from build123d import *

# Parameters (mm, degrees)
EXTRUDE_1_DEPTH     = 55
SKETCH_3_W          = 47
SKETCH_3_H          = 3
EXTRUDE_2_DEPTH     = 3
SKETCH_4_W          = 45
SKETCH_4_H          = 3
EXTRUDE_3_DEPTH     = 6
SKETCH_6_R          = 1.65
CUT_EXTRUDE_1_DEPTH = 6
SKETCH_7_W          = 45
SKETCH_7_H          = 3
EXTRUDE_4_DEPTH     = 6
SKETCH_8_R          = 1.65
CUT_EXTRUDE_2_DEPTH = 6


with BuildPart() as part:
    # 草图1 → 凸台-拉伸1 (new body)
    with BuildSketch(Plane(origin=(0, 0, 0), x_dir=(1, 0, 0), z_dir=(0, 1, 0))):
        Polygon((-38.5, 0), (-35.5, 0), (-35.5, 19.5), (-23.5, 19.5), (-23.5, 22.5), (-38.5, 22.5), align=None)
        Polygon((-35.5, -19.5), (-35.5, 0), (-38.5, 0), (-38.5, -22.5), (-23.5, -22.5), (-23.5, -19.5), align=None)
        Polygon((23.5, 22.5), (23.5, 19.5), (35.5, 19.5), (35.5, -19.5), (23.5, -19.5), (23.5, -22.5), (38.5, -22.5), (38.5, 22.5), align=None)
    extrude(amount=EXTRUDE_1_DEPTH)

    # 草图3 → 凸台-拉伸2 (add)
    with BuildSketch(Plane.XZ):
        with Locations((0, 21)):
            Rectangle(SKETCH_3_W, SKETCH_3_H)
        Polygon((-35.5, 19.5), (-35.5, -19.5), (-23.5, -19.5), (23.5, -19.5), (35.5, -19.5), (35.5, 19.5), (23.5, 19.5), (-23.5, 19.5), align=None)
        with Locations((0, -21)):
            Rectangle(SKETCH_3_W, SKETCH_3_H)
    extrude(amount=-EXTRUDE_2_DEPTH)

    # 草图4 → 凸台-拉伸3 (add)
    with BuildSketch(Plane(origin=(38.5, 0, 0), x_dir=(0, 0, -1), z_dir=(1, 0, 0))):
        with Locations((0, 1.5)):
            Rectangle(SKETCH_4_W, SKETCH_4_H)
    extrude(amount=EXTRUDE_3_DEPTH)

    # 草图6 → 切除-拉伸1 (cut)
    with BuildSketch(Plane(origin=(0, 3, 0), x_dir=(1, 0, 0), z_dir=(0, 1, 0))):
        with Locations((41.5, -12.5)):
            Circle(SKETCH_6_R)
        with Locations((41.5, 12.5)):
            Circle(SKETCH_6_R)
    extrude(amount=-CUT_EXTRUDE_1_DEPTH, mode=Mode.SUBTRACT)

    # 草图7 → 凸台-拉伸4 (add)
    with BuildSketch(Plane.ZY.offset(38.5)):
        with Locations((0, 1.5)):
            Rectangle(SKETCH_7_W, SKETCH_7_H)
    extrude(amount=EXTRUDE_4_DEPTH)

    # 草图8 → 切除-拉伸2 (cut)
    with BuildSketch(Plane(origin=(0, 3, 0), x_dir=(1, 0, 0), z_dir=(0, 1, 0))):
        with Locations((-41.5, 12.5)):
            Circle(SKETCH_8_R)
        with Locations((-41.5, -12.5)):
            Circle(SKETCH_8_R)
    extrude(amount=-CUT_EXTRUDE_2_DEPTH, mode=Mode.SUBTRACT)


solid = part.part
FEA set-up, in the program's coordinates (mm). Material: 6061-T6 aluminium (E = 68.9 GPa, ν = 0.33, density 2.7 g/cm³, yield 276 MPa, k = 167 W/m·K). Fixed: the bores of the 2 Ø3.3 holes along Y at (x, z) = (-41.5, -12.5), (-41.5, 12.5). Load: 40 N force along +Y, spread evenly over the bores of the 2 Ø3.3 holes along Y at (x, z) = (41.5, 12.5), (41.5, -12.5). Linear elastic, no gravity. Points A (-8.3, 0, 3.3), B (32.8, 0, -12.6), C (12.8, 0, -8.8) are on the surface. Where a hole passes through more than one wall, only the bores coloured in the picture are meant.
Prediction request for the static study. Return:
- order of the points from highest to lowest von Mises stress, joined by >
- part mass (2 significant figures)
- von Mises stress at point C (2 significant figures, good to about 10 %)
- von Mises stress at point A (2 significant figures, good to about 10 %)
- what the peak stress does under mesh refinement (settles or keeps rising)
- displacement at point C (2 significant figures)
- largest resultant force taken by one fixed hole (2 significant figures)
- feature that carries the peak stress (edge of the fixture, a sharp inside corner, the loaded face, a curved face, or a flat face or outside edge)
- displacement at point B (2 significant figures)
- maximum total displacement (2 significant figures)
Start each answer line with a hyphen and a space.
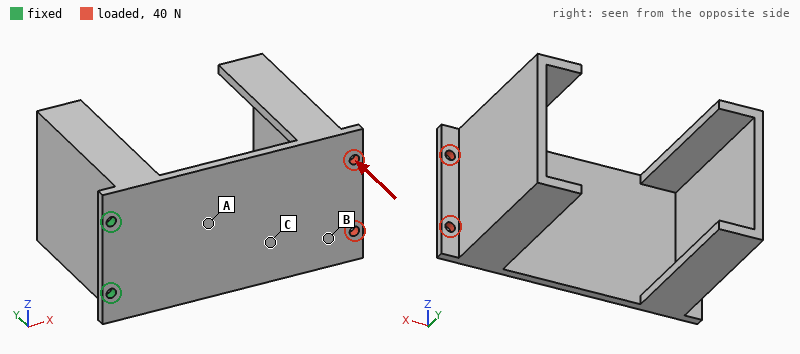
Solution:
- A > C > B
- 90 g
- 17 MPa
- 28 MPa
- keeps rising
- 0.45 mm
- 33 N
- edge of the fixture
- 0.77 mm
- 1.3 mm
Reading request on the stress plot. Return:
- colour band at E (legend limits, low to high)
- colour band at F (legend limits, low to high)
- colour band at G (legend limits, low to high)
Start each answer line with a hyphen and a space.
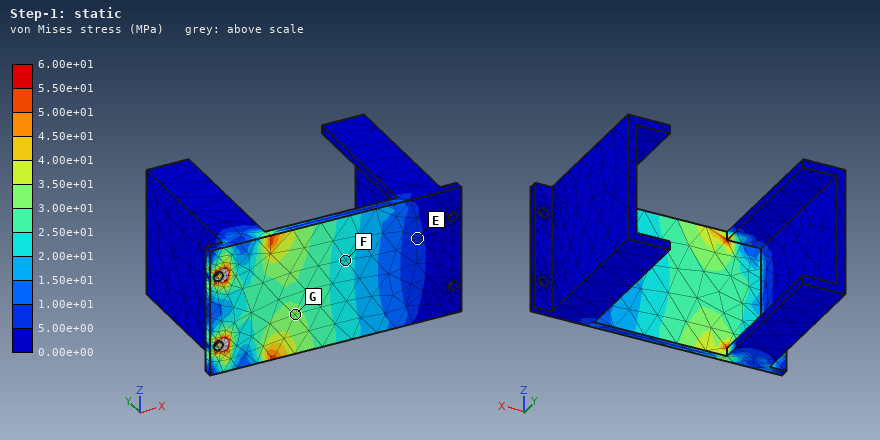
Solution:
- 5.00e+00 to 1.00e+01 MPa
- 2.00e+01 to 2.50e+01 MPa
- 3.00e+01 to 3.50e+01 MPa
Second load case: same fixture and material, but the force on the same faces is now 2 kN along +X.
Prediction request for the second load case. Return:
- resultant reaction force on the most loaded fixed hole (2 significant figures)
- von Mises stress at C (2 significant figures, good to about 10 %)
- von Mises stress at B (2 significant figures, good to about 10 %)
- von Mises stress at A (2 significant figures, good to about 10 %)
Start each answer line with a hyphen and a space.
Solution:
- 1.0 kN
- 15 MPa
- 24 MPa
- 15 MPa
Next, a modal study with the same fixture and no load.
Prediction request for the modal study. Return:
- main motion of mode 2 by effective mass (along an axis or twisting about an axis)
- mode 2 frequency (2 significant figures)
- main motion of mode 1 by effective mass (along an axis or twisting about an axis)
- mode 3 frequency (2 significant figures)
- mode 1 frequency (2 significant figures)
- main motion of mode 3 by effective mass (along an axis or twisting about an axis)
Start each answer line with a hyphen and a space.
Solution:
- along Z
- 400 Hz
- along Y
- 640 Hz
- 170 Hz
- along Y
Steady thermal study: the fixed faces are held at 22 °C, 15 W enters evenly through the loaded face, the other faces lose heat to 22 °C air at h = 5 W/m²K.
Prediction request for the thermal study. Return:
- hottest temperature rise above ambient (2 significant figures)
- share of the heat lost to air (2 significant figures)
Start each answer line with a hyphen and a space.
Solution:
- 51 K
- 18 %
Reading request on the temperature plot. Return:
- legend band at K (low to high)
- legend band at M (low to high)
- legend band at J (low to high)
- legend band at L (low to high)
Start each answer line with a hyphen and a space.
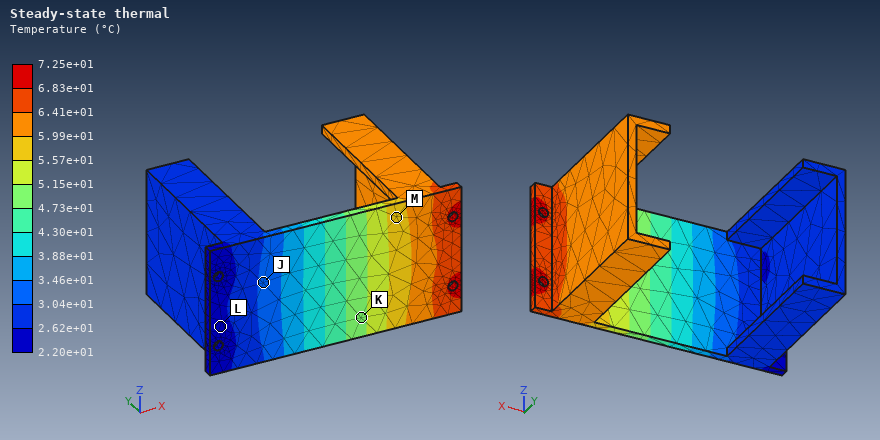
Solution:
- 4.73e+01 to 5.15e+01 °C
- 5.57e+01 to 5.99e+01 °C
- 3.04e+01 to 3.46e+01 °C
- 2.20e+01 to 2.62e+01 °C
